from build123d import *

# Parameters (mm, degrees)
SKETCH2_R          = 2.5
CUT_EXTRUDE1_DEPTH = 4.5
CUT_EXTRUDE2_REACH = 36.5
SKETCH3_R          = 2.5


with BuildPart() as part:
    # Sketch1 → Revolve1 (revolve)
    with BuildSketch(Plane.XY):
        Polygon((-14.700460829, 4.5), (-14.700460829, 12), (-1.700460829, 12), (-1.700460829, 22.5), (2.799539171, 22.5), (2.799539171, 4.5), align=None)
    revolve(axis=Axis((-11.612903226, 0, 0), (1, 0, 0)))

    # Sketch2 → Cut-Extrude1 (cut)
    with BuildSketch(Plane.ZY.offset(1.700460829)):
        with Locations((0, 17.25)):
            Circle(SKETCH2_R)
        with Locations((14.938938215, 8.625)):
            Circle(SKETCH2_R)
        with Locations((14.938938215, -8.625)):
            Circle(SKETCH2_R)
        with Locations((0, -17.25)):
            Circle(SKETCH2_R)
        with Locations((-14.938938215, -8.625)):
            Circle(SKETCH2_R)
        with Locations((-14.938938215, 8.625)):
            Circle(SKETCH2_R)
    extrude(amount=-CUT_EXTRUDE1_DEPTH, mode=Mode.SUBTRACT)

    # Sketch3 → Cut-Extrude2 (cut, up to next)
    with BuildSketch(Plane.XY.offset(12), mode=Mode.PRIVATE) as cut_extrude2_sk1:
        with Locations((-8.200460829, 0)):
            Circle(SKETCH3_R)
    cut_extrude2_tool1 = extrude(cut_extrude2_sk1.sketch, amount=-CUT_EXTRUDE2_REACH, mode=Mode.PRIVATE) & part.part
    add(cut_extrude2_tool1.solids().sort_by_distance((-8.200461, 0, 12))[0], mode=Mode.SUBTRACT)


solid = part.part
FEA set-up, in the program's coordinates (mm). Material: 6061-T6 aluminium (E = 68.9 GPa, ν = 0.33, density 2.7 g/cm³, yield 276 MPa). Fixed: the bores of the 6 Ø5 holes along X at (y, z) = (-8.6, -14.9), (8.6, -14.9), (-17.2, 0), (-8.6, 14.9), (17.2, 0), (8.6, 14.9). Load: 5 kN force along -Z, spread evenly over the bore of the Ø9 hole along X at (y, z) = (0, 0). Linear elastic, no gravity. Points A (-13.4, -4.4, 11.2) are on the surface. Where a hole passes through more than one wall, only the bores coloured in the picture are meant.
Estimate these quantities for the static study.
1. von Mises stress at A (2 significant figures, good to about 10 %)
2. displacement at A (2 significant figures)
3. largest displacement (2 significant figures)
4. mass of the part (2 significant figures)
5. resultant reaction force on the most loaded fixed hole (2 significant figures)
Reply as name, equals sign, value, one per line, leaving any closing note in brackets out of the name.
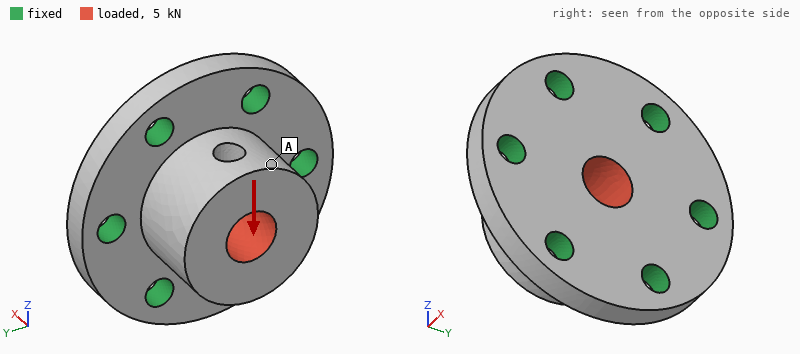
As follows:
von Mises stress at A = 8.3 MPa
displacement at A = 12 µm
largest displacement = 13 µm
mass of the part = 30 g
resultant reaction force on the most loaded fixed hole = 1.3 kN
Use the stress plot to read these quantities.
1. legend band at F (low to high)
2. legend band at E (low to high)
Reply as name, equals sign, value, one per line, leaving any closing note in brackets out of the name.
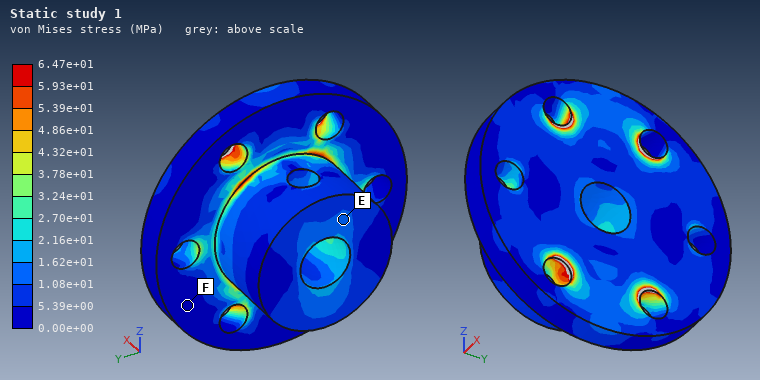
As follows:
legend band at F = 0.00e+00 to 5.39e+00 MPa
legend band at E = 1.08e+01 to 1.62e+01 MPa
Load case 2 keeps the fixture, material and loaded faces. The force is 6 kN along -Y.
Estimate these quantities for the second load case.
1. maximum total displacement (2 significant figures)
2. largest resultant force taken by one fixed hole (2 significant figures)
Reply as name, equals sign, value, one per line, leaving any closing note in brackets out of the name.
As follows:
maximum total displacement = 16 µm
largest resultant force taken by one fixed hole = 1.8 kN
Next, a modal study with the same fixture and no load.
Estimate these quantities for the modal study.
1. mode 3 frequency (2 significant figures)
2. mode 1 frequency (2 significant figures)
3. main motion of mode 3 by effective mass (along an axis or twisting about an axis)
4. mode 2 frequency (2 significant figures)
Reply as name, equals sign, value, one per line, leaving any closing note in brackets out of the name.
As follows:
mode 3 frequency = 31 kHz
mode 1 frequency = 27 kHz
main motion of mode 3 by effective mass = along X
mode 2 frequency = 27 kHz
